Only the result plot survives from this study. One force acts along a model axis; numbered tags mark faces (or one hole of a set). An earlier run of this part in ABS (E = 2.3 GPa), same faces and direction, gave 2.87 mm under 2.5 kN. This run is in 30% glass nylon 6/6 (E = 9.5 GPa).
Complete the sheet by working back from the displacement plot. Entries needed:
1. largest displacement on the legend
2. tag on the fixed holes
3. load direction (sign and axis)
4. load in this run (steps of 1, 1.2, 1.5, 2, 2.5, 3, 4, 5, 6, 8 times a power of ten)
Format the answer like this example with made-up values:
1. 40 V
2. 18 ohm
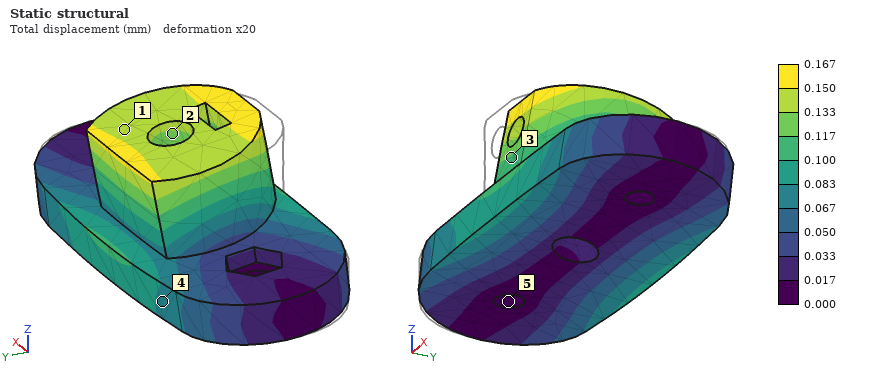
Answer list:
1. 0.167 mm
2. 5
3. +Y
4. 600 N
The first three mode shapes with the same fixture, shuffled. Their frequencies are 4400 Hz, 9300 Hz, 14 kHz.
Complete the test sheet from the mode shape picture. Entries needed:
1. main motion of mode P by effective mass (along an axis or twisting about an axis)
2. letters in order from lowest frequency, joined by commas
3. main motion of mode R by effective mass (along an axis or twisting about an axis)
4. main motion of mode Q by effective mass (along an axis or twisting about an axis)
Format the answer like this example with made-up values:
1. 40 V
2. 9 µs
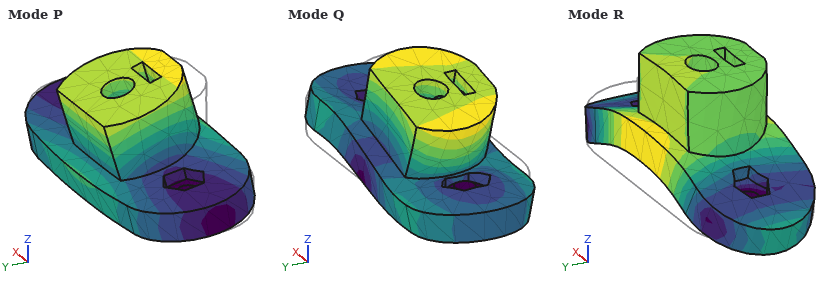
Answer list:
1. along Y
2. P, R, Q
3. along Z
4. along X
